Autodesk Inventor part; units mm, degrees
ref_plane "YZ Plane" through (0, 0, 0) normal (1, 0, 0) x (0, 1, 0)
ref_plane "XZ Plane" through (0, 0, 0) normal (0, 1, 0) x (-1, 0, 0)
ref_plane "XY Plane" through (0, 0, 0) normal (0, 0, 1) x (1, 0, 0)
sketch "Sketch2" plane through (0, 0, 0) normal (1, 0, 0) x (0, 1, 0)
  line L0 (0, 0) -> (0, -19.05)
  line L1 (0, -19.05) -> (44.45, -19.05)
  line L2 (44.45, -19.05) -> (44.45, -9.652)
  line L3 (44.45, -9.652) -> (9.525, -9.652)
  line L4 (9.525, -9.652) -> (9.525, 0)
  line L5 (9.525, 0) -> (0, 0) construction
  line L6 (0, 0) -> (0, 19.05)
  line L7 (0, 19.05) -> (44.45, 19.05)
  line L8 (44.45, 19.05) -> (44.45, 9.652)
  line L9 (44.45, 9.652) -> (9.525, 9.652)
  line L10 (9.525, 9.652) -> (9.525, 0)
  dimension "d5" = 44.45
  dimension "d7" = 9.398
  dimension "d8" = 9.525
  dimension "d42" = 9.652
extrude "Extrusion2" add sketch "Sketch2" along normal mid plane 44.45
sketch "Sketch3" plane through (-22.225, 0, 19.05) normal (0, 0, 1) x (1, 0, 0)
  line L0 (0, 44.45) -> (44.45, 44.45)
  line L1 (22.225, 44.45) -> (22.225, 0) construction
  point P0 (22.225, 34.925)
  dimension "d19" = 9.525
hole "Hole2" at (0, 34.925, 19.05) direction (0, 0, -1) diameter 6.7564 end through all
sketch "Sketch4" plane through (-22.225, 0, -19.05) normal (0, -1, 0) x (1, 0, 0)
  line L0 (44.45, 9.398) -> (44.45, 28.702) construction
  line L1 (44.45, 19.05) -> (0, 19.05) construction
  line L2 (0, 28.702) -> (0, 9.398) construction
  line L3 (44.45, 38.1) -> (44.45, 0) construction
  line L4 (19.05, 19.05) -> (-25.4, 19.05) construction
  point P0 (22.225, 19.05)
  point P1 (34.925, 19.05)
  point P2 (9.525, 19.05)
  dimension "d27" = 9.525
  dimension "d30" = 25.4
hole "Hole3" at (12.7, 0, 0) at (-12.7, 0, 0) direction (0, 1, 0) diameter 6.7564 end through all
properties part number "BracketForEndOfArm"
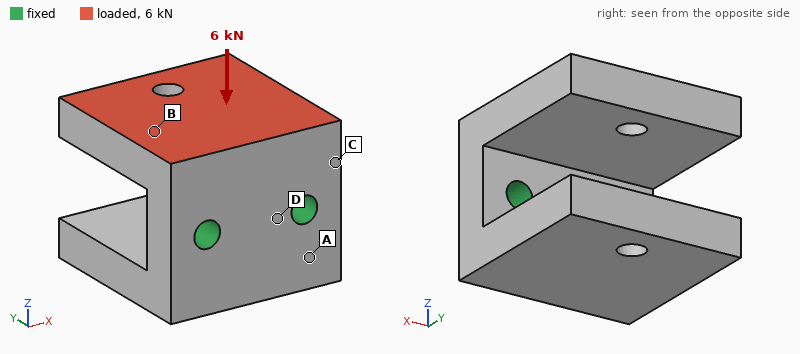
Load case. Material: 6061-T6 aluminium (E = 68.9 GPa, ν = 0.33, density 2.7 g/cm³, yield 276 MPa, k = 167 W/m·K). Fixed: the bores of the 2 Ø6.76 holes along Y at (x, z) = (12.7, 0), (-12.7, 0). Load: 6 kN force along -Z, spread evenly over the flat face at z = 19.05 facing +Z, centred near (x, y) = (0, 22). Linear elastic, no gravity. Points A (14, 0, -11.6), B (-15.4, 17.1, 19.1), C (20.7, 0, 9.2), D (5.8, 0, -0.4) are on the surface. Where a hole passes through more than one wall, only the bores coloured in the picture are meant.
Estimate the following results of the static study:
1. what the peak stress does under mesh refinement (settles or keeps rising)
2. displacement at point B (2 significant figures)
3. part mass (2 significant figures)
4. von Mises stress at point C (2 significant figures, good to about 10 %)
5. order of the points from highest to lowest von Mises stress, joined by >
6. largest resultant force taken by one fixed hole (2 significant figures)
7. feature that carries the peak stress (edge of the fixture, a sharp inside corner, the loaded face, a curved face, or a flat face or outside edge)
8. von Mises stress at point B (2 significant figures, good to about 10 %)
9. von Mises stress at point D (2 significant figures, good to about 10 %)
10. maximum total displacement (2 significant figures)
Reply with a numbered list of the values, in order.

1. keeps rising
2. 0.12 mm
3. 120 g
4. 120 MPa
5. C > B > D > A
6. 3.1 kN
7. edge of the fixture
8. 78 MPa
9. 47 MPa
10. 0.39 mm
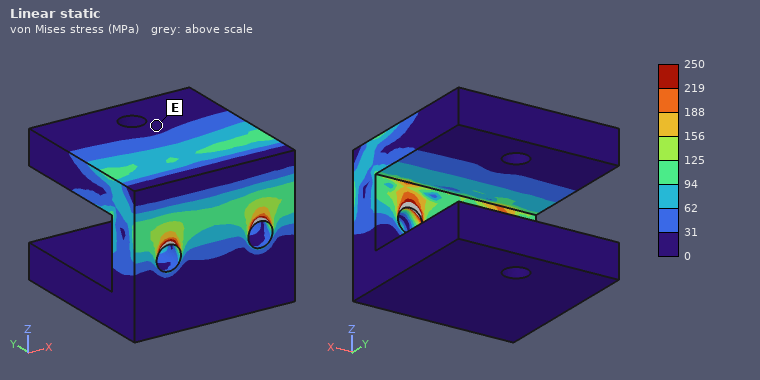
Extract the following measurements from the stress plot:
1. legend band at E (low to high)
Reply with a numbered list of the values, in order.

1. 0 to 31 MPa
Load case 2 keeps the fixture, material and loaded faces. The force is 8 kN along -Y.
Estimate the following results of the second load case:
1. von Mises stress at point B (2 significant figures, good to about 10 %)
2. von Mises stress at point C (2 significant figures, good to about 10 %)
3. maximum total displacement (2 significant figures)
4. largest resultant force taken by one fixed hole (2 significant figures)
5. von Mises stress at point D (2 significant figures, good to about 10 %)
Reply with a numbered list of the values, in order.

1. 48 MPa
2. 98 MPa
3. 0.31 mm
4. 4.0 kN
5. 71 MPa
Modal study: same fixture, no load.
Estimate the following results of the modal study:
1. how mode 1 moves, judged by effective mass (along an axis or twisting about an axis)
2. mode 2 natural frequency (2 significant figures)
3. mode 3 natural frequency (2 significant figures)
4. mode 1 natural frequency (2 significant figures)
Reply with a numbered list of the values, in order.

1. along Z
2. 3500 Hz
3. 6500 Hz
4. 3300 Hz
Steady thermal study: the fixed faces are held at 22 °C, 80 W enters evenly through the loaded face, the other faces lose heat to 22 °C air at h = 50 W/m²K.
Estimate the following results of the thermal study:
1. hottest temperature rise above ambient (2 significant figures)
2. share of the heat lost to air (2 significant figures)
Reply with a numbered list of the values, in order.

1. 31 K
2. 5.6 %
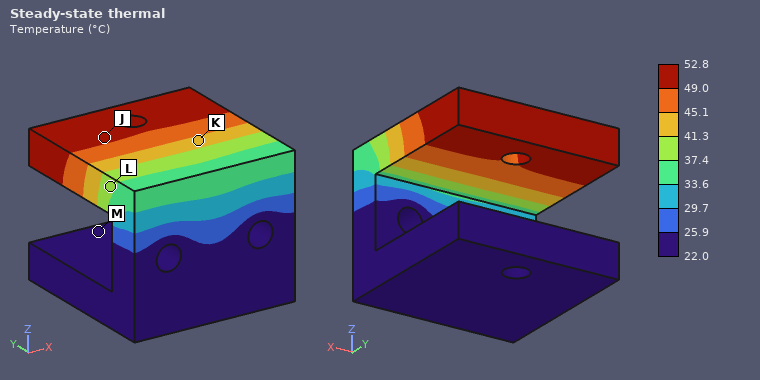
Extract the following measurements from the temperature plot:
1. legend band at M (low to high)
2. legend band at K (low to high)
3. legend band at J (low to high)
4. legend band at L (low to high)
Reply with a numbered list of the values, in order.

1. 22.0 to 25.9 °C
2. 41.3 to 45.1 °C
3. 49.0 to 52.8 °C
4. 37.4 to 41.3 °C
